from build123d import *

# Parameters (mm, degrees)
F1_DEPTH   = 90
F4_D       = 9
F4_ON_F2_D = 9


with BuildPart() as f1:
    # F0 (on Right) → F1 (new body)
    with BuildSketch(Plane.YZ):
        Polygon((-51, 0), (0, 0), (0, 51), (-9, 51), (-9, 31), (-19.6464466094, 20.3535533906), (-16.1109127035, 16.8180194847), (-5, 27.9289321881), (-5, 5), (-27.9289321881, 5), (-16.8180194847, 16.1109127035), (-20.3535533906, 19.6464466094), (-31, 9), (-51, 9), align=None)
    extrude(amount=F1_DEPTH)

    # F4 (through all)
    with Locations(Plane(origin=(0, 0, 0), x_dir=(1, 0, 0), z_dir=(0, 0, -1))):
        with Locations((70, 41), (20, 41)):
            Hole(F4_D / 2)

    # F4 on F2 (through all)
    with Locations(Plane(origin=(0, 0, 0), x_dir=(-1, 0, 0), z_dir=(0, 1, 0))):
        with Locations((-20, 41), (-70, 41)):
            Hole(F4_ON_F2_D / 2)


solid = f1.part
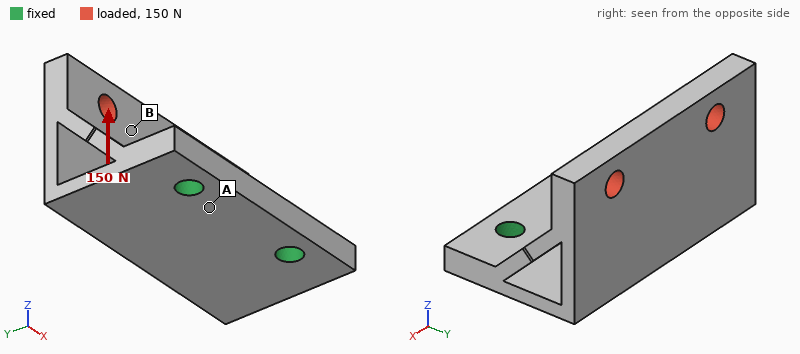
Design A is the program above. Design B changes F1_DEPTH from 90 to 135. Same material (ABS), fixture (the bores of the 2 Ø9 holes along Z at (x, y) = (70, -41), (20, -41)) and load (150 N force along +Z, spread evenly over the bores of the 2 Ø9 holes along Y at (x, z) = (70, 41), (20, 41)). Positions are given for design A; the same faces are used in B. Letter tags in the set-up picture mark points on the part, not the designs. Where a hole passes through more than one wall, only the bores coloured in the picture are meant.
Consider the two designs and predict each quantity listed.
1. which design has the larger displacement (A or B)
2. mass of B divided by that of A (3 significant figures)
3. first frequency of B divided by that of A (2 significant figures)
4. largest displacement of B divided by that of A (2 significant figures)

A
1.52
0.94
0.88
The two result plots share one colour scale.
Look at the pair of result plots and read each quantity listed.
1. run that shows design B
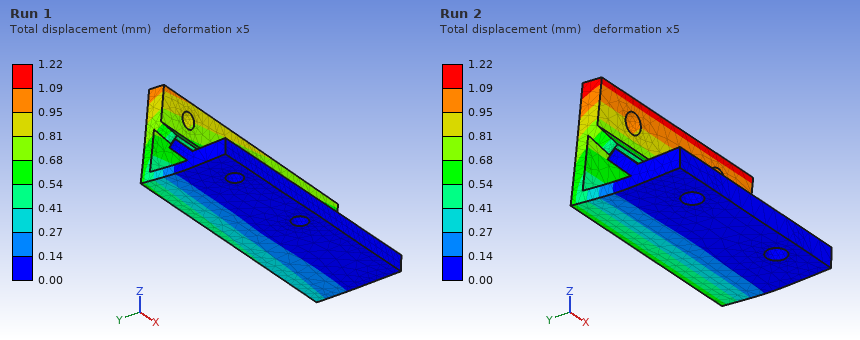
Run 1
